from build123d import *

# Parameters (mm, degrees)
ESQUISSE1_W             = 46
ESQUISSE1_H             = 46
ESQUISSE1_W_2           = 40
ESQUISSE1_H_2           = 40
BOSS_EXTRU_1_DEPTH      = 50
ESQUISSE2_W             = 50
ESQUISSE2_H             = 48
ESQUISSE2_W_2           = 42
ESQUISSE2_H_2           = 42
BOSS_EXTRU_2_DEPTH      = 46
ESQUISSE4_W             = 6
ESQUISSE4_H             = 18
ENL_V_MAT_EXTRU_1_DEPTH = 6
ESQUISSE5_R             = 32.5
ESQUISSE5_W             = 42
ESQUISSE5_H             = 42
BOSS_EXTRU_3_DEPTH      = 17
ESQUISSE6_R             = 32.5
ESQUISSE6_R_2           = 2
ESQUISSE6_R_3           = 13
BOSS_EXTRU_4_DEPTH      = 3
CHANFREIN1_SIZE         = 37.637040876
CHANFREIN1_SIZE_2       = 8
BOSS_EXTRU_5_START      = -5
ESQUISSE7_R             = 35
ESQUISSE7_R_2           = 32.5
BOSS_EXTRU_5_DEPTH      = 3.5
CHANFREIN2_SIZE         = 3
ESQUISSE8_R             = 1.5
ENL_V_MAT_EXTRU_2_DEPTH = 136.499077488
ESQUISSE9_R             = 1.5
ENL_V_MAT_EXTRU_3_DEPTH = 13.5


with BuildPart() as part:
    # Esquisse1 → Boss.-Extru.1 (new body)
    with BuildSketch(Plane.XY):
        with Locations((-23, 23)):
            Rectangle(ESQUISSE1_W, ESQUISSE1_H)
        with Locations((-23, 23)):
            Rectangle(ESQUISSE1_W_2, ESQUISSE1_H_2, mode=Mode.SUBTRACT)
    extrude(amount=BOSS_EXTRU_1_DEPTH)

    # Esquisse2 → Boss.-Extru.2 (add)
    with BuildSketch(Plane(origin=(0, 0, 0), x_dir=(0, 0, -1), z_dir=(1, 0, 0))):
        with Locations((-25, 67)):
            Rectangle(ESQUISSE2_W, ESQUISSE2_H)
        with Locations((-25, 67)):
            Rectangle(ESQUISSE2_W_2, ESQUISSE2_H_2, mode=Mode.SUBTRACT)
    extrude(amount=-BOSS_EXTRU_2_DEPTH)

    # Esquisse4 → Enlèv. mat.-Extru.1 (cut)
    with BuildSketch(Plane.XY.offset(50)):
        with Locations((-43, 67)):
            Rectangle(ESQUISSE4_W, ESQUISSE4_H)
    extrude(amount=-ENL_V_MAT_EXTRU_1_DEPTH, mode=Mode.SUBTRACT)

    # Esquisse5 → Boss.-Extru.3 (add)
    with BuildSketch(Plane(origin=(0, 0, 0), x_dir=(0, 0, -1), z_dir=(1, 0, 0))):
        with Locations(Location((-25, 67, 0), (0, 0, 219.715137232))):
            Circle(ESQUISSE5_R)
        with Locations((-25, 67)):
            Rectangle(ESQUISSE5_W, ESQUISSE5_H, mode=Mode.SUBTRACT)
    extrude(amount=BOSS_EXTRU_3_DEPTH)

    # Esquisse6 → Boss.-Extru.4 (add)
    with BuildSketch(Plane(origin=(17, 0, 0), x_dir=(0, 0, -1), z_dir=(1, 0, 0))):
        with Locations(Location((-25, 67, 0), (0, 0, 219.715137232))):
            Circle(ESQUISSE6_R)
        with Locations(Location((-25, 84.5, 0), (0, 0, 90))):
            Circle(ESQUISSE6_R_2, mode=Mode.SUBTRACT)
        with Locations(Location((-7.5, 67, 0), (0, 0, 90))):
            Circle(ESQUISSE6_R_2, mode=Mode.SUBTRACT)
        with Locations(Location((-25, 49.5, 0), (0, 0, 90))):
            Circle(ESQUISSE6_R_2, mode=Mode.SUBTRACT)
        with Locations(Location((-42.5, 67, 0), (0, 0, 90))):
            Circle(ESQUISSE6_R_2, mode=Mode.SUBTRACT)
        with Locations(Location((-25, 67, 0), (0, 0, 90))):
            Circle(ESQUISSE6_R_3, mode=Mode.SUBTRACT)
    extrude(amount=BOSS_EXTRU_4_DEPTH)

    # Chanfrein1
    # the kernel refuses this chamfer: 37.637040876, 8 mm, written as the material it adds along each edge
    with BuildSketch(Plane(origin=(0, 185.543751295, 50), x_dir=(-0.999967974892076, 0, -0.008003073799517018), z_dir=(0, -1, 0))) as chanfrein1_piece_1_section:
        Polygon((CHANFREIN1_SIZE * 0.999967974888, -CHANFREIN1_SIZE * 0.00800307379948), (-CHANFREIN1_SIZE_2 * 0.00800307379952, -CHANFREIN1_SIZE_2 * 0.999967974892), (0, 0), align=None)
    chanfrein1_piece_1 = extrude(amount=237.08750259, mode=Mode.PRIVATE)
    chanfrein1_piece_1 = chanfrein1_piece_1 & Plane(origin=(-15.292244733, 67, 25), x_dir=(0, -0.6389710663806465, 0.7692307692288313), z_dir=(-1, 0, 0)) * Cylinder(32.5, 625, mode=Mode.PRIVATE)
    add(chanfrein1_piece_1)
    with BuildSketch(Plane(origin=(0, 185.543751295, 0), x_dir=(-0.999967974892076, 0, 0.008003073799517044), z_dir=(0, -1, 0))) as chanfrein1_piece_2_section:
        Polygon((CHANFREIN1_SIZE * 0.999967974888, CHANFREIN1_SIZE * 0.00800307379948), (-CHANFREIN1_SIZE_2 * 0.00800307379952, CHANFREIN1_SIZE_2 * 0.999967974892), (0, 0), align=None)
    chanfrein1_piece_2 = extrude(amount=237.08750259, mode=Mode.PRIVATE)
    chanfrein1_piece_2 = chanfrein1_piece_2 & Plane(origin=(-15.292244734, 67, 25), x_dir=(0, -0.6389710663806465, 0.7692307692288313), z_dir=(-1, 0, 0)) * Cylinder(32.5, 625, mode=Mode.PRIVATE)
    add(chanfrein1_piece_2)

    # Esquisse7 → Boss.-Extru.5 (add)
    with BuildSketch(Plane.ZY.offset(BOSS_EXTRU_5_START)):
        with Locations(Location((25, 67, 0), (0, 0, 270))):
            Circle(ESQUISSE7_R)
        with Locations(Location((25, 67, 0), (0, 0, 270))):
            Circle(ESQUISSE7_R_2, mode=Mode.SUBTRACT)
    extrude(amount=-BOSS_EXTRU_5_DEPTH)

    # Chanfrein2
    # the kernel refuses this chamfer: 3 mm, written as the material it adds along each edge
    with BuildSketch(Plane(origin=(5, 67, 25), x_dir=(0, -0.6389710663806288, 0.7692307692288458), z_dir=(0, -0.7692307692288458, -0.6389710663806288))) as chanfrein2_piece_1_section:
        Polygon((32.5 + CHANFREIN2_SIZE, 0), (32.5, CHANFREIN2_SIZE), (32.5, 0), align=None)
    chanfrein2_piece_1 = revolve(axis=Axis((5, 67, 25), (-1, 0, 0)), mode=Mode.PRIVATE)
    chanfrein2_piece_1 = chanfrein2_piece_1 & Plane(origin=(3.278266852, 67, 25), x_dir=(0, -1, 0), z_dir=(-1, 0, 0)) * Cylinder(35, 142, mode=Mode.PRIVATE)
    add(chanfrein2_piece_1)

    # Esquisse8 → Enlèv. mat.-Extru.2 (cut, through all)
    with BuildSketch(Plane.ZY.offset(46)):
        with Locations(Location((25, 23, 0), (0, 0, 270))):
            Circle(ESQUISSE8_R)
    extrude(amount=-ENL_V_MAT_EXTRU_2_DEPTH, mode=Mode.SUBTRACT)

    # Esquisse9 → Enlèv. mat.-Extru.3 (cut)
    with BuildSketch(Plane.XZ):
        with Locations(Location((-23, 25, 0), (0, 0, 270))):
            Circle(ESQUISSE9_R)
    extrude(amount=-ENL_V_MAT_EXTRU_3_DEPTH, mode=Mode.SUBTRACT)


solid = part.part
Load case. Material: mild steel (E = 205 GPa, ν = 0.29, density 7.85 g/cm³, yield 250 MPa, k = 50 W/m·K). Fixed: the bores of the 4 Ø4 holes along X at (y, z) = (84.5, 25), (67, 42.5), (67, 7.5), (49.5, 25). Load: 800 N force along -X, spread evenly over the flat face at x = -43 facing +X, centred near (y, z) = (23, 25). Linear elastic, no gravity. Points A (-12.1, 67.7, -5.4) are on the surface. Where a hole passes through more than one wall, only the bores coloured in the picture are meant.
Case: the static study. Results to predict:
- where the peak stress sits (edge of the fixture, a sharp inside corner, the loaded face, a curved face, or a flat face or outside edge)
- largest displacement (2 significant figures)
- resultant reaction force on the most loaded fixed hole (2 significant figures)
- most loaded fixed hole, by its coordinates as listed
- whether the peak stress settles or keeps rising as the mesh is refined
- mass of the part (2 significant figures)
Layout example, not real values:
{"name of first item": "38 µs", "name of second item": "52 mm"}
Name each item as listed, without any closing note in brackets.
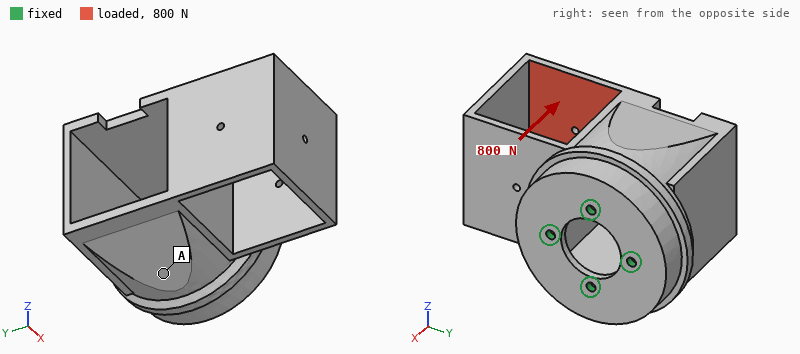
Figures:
{"where the peak stress sits": "edge of the fixture", "largest displacement": "73 µm", "resultant reaction force on the most loaded fixed hole": "1.1 kN", "most loaded fixed hole, by its coordinates as listed": "(49.5, 25)", "whether the peak stress settles or keeps rising as the mesh is refined": "keeps rising", "mass of the part": "750 g"}
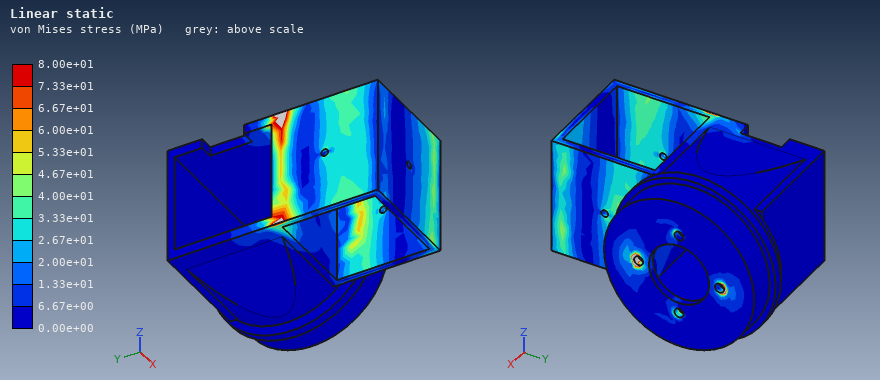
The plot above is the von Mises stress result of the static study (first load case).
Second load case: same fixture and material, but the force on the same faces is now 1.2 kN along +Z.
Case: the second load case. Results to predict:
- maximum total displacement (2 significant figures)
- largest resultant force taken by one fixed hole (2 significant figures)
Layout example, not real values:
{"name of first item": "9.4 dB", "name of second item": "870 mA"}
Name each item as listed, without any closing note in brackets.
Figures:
{"maximum total displacement": "43 µm", "largest resultant force taken by one fixed hole": "1.9 kN"}
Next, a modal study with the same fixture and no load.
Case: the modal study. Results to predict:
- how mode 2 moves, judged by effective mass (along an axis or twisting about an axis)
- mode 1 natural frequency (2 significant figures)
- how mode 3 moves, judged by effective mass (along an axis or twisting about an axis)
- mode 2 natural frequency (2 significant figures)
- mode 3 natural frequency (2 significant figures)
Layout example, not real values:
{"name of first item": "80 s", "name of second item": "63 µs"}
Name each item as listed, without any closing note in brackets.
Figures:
{"how mode 2 moves, judged by effective mass": "along Z", "mode 1 natural frequency": "1300 Hz", "how mode 3 moves, judged by effective mass": "along Y", "mode 2 natural frequency": "2000 Hz", "mode 3 natural frequency": "2300 Hz"}
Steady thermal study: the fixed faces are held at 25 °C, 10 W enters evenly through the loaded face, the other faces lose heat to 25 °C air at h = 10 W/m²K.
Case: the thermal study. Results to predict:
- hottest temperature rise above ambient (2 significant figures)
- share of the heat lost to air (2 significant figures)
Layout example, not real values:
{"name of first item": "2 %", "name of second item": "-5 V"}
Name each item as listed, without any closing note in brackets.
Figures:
{"hottest temperature rise above ambient": "32 K", "share of the heat lost to air": "39 %"}
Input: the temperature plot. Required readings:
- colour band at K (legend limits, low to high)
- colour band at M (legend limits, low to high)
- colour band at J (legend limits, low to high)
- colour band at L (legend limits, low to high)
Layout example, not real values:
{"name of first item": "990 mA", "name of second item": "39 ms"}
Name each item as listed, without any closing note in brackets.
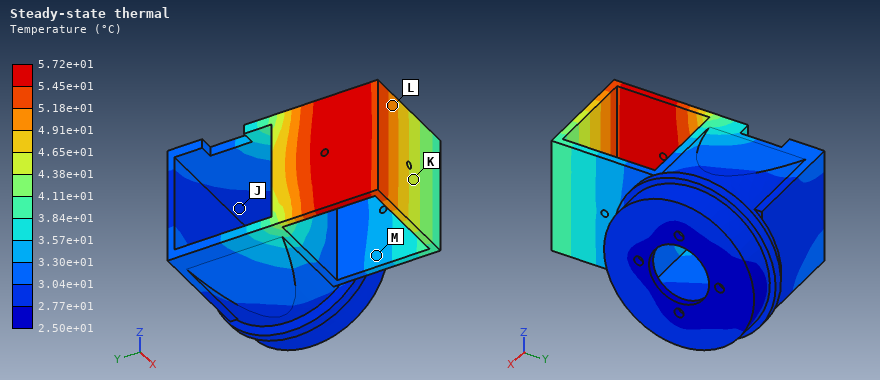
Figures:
{"colour band at K": "4.38e+01 to 4.65e+01 °C", "colour band at M": "3.30e+01 to 3.57e+01 °C", "colour band at J": "2.77e+01 to 3.04e+01 °C", "colour band at L": "4.91e+01 to 5.18e+01 °C"}
